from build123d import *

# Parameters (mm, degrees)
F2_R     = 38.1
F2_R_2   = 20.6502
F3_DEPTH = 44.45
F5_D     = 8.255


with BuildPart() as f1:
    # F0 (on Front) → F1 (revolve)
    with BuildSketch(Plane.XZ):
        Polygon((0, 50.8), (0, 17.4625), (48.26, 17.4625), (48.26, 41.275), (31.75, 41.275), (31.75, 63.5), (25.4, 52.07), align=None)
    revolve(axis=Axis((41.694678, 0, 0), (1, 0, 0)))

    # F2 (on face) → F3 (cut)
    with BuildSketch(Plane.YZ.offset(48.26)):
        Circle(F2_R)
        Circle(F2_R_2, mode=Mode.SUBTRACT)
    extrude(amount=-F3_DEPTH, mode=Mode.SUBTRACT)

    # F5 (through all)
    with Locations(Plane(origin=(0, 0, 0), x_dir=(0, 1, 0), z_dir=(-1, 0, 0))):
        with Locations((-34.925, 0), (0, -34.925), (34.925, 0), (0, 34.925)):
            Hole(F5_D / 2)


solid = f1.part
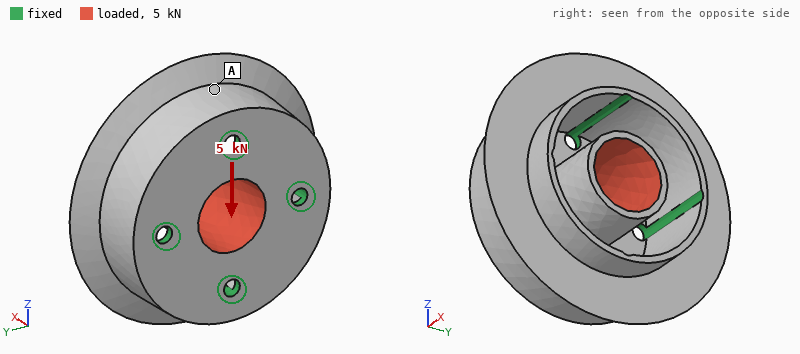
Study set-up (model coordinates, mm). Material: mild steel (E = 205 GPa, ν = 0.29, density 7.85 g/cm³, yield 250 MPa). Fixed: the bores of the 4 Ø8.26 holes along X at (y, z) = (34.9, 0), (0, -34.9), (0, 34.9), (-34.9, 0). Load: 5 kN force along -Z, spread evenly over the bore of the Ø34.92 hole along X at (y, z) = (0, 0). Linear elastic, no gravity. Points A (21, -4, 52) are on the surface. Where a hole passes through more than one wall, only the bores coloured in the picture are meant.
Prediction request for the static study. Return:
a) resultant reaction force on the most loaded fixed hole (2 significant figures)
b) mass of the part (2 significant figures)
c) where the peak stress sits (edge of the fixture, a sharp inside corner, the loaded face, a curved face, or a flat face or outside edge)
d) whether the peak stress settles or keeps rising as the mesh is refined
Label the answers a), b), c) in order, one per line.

a) 2.4 kN
b) 1.4 kg
c) edge of the fixture
d) keeps rising
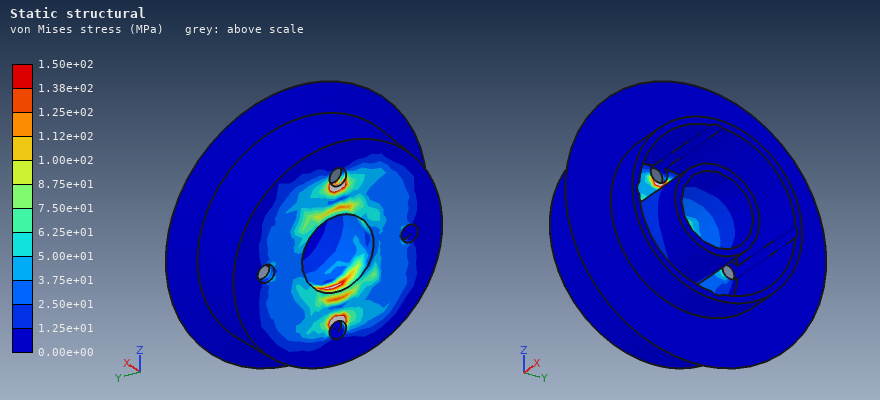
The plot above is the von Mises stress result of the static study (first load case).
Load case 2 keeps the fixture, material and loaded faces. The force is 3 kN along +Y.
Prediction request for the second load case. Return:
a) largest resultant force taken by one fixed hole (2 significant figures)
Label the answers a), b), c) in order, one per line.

a) 1.4 kN
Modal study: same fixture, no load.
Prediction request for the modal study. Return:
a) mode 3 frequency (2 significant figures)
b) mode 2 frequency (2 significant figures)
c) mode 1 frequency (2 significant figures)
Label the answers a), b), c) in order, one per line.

a) 6700 Hz
b) 4400 Hz
c) 4400 Hz
